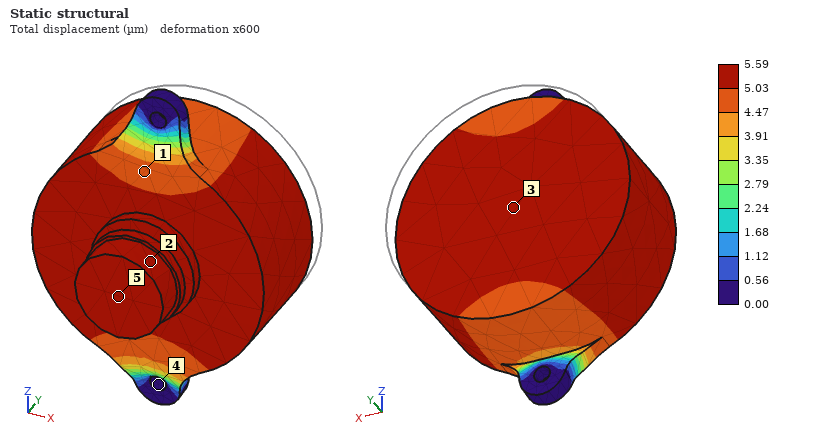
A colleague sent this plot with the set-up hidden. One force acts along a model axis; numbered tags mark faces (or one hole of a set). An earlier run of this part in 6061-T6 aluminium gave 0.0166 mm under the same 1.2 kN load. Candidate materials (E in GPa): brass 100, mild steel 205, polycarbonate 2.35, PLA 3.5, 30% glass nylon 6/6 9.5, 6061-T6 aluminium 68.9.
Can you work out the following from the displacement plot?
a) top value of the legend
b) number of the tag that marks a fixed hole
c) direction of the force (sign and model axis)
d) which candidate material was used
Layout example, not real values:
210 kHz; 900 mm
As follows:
5.59 µm; 4; -Y; mild steel
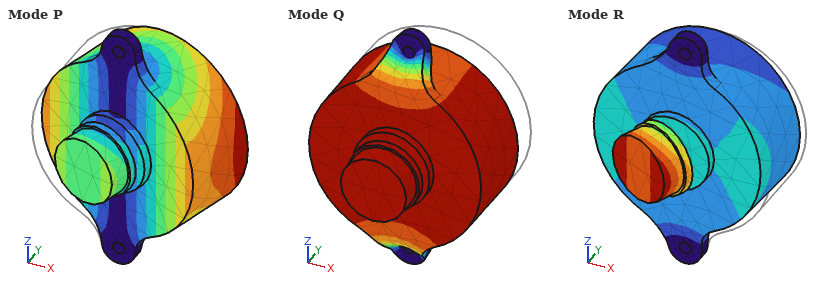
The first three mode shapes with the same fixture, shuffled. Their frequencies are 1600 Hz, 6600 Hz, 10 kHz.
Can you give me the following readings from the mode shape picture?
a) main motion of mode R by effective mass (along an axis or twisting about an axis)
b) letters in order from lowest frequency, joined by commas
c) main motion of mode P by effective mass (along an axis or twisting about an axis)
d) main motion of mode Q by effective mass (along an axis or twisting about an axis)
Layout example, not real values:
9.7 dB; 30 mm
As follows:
along X; P, Q, R; along X; along Y
